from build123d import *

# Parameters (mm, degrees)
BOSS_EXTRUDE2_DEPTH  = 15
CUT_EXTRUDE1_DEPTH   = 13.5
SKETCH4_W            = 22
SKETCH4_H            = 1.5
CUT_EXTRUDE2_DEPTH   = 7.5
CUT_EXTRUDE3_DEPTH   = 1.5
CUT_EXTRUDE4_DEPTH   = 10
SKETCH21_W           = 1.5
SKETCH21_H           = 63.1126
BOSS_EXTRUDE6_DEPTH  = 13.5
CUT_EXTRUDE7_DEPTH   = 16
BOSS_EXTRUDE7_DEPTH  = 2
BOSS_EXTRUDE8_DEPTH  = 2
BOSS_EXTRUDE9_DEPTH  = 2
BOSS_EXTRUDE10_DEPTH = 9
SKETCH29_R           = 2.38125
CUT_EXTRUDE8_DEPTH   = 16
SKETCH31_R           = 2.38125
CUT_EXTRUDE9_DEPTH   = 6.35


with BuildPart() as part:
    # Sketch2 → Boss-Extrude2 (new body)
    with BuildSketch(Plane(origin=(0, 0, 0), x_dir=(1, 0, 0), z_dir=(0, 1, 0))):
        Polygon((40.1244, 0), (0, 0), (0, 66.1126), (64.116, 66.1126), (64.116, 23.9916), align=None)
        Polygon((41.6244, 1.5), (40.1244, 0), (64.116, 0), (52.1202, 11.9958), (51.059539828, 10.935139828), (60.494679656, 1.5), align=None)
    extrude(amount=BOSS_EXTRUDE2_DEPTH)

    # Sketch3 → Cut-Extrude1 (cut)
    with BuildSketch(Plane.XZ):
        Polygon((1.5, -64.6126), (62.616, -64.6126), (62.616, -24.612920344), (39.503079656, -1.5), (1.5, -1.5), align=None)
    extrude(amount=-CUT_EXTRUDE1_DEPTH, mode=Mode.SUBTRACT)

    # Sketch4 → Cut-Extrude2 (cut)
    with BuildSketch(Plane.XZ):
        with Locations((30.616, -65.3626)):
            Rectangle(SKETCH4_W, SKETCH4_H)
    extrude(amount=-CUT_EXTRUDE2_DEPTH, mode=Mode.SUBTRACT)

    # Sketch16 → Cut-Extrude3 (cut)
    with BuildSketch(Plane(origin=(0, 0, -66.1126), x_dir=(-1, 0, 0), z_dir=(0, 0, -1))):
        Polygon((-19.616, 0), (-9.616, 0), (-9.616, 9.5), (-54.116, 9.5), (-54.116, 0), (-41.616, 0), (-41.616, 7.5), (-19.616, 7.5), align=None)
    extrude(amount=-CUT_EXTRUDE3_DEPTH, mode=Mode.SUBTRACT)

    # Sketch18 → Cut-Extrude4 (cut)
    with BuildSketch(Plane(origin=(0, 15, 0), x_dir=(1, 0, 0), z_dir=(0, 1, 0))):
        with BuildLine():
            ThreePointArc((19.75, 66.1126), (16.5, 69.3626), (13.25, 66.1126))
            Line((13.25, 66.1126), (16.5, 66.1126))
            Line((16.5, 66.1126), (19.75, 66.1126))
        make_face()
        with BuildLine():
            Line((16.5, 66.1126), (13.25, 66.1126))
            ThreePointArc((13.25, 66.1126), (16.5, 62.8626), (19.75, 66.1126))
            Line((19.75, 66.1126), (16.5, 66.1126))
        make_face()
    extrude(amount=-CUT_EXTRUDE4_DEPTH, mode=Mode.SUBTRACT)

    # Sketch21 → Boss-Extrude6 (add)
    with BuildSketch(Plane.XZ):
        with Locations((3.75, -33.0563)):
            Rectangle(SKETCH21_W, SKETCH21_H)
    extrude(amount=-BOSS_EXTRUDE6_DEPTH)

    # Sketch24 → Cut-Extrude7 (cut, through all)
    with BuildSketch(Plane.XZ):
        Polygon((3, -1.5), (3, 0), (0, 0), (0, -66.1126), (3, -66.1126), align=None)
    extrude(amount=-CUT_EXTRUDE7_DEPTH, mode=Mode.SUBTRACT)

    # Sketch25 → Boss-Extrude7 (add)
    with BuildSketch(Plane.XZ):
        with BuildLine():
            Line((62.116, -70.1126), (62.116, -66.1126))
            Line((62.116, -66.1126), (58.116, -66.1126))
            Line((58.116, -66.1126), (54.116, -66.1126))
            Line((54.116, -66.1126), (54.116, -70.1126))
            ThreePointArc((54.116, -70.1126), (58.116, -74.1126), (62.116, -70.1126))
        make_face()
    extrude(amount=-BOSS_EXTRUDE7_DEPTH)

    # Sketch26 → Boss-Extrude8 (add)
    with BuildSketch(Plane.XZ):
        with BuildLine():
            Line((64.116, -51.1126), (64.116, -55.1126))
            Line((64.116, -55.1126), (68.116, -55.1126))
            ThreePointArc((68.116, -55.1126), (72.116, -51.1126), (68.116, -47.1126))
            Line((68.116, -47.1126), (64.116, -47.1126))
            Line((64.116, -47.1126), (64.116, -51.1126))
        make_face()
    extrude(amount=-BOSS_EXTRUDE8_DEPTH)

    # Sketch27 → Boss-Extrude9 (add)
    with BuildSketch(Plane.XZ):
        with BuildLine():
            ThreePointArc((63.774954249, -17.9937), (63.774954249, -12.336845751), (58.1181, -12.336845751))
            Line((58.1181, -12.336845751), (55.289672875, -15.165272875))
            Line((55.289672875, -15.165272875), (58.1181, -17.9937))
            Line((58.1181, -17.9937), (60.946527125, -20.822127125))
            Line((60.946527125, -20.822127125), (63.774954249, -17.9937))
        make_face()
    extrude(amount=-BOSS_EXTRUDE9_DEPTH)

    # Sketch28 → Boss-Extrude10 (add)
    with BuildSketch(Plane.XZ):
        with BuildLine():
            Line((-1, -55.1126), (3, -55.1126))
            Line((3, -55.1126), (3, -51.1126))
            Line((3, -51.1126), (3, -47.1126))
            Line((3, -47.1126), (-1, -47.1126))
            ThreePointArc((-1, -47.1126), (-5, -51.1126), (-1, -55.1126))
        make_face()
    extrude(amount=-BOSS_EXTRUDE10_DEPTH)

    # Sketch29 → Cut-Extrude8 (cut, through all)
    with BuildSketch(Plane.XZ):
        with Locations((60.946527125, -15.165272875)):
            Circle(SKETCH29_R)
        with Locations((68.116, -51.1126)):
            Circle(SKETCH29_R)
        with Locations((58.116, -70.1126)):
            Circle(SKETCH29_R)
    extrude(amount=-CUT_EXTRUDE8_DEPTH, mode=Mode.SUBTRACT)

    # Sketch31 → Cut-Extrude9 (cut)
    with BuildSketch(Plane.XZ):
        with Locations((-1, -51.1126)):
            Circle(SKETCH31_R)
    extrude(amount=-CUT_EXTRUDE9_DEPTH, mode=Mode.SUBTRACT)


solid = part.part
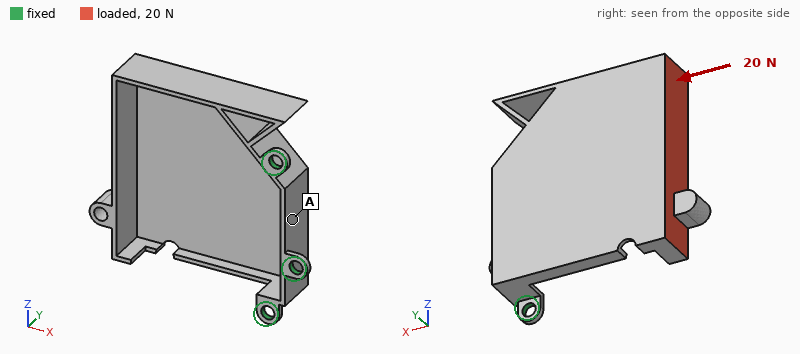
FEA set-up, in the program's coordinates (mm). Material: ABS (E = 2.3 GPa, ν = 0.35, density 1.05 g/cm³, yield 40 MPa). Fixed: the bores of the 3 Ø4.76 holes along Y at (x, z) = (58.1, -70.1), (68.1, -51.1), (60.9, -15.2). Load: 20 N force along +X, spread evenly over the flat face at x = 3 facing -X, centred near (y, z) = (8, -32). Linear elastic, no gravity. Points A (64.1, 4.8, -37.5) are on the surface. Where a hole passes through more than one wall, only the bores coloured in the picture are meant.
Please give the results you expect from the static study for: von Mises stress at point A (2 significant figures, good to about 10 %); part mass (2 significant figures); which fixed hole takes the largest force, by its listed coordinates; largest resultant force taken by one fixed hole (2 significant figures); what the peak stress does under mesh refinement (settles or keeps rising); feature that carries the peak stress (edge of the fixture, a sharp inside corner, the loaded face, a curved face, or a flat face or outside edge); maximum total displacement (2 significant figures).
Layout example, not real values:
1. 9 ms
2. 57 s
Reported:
1. 0.77 MPa
2. 12 g
3. (60.9, -15.2)
4. 14 N
5. keeps rising
6. edge of the fixture
7. 1.1 mm
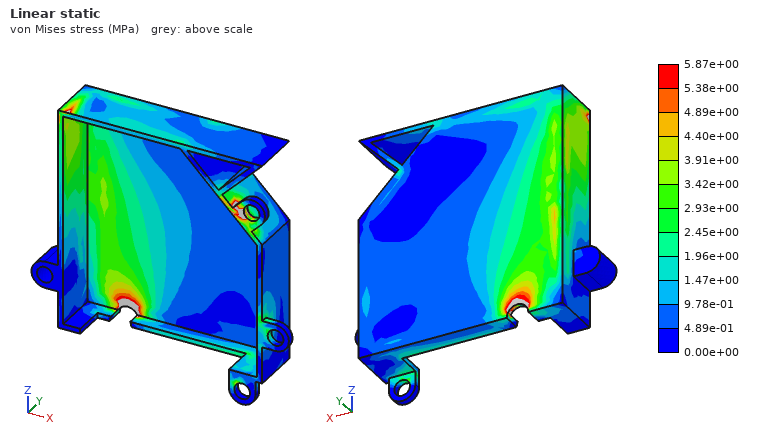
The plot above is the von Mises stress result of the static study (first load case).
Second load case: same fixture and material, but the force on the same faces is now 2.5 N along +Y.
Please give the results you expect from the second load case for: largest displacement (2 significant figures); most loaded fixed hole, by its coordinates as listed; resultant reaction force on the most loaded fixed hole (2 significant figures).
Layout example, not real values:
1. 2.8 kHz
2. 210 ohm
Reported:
1. 1.1 mm
2. (68.1, -51.1)
3. 10 N
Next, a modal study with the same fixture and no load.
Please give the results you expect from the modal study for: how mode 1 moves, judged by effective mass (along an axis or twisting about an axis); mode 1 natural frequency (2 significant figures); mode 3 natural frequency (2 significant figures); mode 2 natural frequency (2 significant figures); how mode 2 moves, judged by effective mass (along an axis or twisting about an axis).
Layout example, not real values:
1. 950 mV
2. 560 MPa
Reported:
1. along Y
2. 130 Hz
3. 460 Hz
4. 200 Hz
5. along Z
